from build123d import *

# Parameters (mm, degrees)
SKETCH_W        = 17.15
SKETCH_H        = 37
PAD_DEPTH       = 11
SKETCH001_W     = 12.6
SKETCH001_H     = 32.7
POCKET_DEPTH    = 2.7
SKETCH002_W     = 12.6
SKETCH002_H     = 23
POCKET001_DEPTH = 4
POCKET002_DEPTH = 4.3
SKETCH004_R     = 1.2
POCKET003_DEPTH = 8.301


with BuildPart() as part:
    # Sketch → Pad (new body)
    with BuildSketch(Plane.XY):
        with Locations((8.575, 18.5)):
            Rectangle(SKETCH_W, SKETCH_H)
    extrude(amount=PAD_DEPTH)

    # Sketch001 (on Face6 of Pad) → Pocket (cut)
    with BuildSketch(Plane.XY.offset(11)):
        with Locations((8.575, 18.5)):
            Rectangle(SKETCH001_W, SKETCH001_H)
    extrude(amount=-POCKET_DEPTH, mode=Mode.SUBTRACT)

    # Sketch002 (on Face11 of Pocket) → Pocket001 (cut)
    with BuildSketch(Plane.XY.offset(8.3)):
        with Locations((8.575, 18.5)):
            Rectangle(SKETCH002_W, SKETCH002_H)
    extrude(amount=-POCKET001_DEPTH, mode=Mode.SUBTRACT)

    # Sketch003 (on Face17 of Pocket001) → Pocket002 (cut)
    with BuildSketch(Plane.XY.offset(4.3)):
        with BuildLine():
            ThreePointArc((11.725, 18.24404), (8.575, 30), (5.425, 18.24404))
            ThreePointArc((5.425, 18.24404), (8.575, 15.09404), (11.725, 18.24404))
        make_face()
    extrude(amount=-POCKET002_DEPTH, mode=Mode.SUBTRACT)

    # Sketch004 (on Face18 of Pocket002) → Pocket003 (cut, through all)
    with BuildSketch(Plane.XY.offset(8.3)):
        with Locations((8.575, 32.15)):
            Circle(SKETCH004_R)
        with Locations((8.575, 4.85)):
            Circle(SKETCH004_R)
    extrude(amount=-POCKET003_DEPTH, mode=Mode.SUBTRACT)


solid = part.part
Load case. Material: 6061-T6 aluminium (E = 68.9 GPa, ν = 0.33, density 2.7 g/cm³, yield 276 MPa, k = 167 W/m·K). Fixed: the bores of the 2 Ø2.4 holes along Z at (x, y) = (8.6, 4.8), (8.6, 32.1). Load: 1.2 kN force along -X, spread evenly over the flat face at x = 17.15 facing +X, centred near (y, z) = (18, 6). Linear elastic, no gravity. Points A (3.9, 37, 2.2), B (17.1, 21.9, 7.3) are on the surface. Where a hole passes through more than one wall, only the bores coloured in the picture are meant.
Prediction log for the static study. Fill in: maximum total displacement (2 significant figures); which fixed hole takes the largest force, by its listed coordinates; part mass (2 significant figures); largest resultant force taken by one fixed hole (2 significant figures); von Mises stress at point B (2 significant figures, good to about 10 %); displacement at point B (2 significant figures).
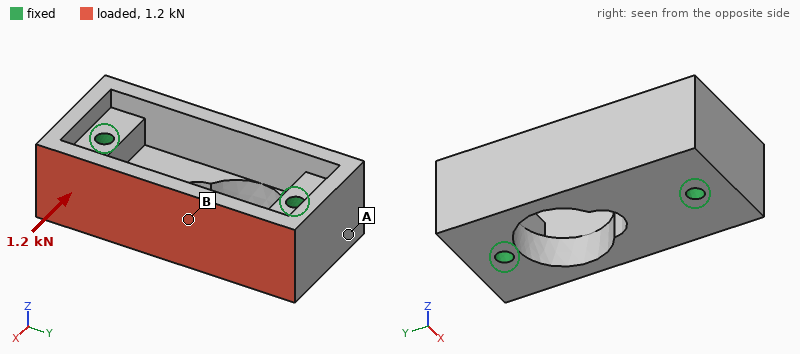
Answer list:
32 µm
(8.6, 4.8)
11 g
680 N
38 MPa
20 µm
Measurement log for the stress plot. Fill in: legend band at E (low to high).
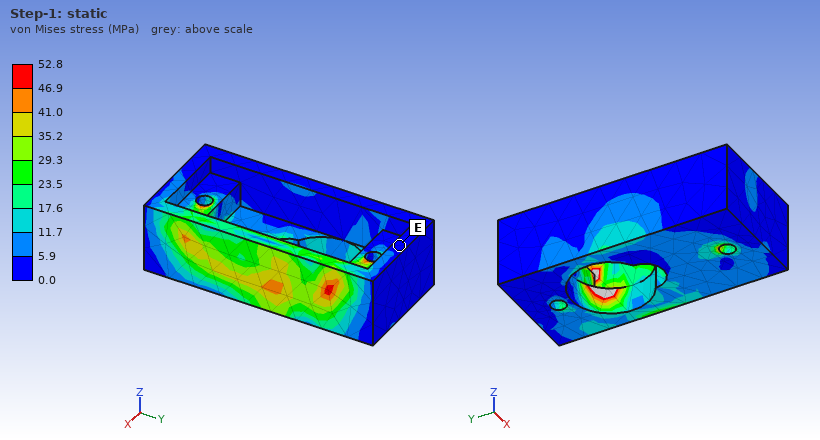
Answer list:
0.0 to 5.9 MPa
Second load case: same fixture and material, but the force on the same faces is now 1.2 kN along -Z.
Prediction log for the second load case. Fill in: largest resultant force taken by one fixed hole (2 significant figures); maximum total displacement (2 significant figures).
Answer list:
620 N
28 µm
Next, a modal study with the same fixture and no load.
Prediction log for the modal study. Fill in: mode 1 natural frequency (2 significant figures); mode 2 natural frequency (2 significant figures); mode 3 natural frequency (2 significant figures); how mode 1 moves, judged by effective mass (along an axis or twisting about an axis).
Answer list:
22 kHz
26 kHz
27 kHz
along X
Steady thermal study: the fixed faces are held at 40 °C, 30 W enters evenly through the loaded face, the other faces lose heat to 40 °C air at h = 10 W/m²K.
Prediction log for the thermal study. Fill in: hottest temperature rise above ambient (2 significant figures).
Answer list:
18 K
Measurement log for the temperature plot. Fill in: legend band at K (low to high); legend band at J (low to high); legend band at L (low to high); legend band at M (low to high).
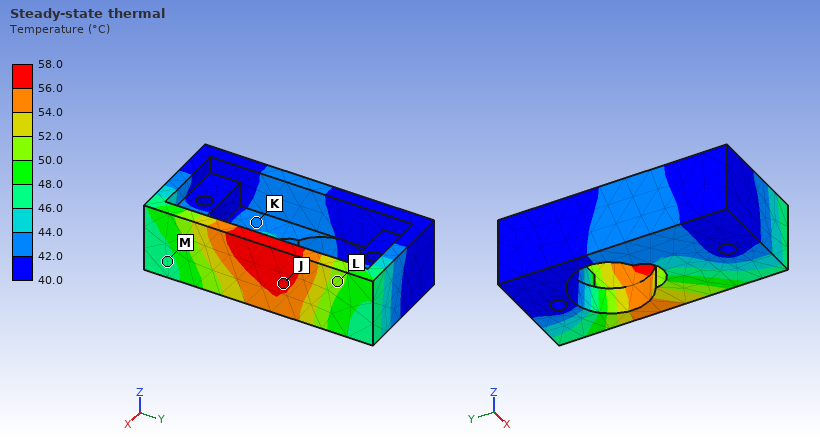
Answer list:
42.0 to 44.0 °C
56.0 to 58.0 °C
50.0 to 52.0 °C
46.0 to 48.0 °C
